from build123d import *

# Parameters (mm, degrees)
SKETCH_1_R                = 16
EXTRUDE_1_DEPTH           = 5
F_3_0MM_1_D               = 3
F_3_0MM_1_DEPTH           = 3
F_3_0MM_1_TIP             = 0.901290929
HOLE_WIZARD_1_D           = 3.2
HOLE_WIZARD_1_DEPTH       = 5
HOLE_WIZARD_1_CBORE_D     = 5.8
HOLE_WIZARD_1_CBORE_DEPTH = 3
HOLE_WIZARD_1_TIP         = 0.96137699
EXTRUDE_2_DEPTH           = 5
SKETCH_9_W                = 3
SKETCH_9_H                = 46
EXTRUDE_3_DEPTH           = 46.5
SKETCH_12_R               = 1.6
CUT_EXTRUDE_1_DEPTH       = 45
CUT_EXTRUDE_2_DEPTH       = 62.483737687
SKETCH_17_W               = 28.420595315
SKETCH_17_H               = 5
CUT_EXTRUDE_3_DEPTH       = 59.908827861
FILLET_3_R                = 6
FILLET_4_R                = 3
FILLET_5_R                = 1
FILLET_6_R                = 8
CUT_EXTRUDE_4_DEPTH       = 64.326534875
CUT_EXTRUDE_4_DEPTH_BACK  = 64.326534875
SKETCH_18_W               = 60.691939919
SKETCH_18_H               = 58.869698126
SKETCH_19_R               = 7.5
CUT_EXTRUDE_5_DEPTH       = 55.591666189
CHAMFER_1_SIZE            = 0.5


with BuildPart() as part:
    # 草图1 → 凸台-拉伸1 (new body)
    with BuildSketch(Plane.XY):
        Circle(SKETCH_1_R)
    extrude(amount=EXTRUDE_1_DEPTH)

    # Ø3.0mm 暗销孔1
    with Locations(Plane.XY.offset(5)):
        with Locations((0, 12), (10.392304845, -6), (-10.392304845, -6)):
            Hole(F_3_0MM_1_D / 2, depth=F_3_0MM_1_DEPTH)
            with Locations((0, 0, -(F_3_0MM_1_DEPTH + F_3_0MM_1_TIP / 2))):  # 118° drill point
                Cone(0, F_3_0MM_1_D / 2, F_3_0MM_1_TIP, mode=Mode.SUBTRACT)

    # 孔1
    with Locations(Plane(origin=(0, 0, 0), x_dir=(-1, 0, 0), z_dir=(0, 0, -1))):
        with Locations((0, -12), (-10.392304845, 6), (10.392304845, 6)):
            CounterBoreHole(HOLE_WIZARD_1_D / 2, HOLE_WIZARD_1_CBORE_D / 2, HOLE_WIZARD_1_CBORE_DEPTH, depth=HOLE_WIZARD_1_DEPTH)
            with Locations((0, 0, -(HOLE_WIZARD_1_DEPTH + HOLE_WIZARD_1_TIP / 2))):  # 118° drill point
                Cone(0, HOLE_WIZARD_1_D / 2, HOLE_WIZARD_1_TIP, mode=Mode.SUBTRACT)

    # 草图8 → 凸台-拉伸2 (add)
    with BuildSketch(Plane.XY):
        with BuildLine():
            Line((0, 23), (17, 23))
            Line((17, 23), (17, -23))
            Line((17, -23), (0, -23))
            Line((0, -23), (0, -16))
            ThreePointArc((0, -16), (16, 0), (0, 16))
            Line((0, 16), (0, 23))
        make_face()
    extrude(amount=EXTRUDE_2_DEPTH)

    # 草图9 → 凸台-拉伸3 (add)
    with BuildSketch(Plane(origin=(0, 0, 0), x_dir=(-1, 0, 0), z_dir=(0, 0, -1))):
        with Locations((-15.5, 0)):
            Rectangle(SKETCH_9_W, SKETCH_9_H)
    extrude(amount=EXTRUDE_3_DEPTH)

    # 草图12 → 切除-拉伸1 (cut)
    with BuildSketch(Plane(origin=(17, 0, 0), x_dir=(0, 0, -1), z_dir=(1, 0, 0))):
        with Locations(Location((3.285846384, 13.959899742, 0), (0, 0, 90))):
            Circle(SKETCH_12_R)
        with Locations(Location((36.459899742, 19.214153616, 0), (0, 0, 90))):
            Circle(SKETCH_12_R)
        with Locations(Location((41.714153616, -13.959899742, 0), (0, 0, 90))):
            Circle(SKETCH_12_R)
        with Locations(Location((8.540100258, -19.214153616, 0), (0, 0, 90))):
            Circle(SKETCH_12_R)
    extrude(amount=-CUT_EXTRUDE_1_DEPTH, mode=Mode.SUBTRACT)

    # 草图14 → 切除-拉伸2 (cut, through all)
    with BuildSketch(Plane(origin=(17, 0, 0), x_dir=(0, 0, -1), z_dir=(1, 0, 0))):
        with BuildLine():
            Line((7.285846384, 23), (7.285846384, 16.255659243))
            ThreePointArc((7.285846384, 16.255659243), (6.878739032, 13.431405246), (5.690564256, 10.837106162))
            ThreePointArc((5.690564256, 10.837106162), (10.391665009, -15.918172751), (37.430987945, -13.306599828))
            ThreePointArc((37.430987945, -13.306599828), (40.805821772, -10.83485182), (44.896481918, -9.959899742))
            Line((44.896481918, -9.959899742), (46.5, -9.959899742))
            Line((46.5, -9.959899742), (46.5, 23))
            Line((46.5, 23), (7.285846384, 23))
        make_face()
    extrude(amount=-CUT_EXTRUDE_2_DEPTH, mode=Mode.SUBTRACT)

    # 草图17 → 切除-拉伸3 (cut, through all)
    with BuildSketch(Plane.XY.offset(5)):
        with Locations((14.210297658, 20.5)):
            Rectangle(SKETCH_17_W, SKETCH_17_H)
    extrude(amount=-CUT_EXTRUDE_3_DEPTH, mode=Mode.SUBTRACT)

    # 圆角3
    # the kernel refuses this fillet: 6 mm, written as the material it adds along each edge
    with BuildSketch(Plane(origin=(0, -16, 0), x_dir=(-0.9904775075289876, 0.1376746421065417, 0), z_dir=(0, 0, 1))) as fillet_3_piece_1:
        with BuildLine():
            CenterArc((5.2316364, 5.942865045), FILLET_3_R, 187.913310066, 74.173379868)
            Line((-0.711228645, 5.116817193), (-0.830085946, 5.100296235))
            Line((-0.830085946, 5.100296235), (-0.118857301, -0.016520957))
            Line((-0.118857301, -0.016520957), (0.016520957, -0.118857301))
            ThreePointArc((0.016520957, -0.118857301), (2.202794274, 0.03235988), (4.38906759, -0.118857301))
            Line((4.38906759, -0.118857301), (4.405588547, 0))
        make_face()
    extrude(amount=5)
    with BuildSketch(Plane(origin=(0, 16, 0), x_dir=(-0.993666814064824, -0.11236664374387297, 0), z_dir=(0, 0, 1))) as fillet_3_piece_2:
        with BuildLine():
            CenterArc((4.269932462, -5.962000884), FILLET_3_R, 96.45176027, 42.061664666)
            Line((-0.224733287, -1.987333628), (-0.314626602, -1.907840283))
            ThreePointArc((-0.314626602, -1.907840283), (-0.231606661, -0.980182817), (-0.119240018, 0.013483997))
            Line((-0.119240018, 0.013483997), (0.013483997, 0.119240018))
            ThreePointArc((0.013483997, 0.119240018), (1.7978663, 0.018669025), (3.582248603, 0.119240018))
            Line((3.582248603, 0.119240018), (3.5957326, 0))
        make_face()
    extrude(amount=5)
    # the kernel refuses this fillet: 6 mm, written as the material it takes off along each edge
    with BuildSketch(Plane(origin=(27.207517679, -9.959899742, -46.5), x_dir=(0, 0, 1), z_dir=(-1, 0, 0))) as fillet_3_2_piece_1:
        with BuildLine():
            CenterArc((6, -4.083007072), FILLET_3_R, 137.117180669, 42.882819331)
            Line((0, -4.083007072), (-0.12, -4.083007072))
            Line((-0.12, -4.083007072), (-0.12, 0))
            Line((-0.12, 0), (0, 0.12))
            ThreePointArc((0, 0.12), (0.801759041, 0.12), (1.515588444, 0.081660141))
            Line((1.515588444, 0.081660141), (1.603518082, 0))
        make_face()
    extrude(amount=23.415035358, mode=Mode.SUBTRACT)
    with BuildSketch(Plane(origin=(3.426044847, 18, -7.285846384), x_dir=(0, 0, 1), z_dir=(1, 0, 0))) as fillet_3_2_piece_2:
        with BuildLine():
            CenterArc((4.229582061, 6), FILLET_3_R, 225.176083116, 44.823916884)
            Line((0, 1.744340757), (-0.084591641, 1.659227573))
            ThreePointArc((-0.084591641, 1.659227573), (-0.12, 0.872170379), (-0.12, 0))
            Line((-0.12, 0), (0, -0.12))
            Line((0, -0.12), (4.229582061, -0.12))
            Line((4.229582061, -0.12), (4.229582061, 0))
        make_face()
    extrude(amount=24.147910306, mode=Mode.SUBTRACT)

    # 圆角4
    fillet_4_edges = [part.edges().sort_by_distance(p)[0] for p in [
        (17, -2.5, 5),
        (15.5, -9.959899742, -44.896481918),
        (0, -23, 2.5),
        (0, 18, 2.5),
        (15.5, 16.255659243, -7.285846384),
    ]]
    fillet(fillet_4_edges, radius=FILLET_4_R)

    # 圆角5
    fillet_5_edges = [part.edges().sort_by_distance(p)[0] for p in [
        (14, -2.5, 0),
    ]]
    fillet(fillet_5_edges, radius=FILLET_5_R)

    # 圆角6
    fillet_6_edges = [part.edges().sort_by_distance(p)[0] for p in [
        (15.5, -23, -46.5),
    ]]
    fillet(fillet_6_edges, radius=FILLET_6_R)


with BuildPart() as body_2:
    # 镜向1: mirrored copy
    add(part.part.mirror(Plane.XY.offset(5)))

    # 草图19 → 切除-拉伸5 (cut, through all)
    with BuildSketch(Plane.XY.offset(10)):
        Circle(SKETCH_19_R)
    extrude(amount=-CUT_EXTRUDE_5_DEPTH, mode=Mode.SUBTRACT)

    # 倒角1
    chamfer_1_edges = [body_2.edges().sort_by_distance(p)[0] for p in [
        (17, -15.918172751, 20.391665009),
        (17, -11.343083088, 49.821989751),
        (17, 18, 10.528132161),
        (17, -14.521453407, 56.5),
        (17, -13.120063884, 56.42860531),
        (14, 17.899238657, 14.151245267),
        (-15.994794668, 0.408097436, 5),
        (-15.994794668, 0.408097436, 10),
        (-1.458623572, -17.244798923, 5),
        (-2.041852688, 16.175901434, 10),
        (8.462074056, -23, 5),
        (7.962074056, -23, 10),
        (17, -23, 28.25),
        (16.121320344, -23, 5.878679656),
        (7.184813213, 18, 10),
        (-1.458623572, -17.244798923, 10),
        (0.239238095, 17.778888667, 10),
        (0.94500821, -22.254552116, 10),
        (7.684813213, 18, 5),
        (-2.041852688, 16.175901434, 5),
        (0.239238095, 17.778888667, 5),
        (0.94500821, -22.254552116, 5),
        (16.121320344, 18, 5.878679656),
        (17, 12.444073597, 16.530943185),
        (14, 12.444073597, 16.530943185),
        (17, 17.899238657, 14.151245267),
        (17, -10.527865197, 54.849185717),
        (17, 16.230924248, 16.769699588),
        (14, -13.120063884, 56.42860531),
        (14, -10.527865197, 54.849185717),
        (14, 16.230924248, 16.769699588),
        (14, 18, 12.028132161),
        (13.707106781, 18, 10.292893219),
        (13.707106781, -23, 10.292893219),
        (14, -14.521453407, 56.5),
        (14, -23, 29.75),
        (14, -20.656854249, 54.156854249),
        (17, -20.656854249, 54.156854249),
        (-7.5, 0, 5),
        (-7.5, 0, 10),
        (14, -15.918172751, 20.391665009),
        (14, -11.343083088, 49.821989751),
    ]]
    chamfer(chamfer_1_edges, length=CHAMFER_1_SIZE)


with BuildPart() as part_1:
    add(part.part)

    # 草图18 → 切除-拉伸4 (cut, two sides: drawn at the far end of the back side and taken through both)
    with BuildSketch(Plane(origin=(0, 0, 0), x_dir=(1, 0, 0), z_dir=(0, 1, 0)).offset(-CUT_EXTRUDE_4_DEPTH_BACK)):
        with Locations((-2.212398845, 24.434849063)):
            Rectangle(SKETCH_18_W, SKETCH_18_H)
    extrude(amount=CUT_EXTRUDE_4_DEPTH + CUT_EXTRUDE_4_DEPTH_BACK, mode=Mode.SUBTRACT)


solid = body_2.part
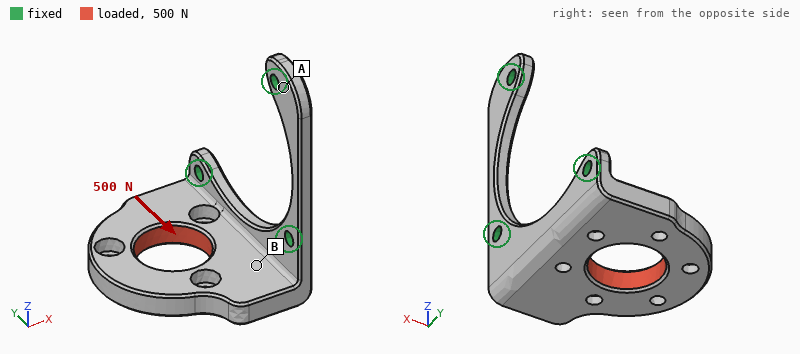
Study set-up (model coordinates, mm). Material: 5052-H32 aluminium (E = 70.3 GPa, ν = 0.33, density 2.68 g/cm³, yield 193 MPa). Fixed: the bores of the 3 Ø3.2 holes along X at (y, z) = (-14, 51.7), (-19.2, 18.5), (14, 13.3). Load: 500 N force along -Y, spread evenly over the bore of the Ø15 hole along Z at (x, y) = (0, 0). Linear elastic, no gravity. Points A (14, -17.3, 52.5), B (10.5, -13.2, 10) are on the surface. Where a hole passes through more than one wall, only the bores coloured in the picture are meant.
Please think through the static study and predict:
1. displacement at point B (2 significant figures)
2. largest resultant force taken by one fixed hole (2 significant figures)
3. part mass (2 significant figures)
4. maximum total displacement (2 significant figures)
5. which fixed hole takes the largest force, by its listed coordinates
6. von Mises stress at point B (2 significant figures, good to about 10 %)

20 µm
400 N
15 g
59 µm
(14, 13.3)
16 MPa
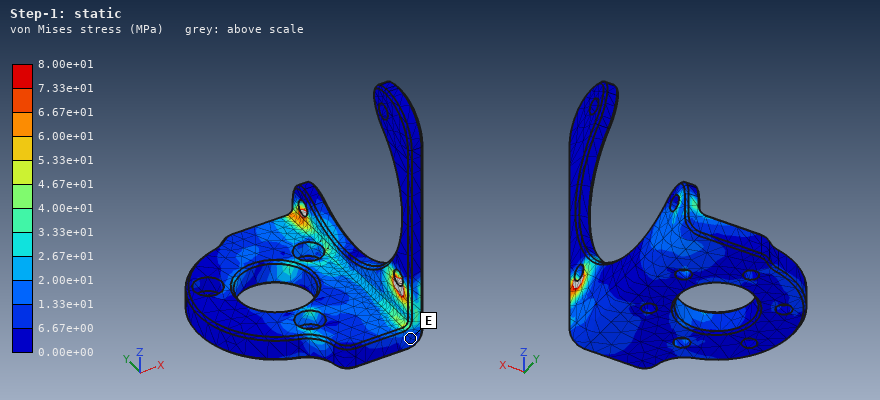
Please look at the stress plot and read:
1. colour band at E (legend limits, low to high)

6.67e+00 to 1.33e+01 MPa
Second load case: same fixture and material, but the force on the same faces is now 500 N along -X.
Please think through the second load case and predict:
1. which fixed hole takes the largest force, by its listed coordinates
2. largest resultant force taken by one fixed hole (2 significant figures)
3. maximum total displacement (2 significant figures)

(14, 13.3)
310 N
0.12 mm
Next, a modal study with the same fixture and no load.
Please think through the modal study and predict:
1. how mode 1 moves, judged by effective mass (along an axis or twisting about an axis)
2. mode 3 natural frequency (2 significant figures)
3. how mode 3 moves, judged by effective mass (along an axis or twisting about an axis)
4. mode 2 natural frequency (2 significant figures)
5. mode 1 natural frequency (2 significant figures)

along Z
9900 Hz
along X
6300 Hz
2200 Hz
